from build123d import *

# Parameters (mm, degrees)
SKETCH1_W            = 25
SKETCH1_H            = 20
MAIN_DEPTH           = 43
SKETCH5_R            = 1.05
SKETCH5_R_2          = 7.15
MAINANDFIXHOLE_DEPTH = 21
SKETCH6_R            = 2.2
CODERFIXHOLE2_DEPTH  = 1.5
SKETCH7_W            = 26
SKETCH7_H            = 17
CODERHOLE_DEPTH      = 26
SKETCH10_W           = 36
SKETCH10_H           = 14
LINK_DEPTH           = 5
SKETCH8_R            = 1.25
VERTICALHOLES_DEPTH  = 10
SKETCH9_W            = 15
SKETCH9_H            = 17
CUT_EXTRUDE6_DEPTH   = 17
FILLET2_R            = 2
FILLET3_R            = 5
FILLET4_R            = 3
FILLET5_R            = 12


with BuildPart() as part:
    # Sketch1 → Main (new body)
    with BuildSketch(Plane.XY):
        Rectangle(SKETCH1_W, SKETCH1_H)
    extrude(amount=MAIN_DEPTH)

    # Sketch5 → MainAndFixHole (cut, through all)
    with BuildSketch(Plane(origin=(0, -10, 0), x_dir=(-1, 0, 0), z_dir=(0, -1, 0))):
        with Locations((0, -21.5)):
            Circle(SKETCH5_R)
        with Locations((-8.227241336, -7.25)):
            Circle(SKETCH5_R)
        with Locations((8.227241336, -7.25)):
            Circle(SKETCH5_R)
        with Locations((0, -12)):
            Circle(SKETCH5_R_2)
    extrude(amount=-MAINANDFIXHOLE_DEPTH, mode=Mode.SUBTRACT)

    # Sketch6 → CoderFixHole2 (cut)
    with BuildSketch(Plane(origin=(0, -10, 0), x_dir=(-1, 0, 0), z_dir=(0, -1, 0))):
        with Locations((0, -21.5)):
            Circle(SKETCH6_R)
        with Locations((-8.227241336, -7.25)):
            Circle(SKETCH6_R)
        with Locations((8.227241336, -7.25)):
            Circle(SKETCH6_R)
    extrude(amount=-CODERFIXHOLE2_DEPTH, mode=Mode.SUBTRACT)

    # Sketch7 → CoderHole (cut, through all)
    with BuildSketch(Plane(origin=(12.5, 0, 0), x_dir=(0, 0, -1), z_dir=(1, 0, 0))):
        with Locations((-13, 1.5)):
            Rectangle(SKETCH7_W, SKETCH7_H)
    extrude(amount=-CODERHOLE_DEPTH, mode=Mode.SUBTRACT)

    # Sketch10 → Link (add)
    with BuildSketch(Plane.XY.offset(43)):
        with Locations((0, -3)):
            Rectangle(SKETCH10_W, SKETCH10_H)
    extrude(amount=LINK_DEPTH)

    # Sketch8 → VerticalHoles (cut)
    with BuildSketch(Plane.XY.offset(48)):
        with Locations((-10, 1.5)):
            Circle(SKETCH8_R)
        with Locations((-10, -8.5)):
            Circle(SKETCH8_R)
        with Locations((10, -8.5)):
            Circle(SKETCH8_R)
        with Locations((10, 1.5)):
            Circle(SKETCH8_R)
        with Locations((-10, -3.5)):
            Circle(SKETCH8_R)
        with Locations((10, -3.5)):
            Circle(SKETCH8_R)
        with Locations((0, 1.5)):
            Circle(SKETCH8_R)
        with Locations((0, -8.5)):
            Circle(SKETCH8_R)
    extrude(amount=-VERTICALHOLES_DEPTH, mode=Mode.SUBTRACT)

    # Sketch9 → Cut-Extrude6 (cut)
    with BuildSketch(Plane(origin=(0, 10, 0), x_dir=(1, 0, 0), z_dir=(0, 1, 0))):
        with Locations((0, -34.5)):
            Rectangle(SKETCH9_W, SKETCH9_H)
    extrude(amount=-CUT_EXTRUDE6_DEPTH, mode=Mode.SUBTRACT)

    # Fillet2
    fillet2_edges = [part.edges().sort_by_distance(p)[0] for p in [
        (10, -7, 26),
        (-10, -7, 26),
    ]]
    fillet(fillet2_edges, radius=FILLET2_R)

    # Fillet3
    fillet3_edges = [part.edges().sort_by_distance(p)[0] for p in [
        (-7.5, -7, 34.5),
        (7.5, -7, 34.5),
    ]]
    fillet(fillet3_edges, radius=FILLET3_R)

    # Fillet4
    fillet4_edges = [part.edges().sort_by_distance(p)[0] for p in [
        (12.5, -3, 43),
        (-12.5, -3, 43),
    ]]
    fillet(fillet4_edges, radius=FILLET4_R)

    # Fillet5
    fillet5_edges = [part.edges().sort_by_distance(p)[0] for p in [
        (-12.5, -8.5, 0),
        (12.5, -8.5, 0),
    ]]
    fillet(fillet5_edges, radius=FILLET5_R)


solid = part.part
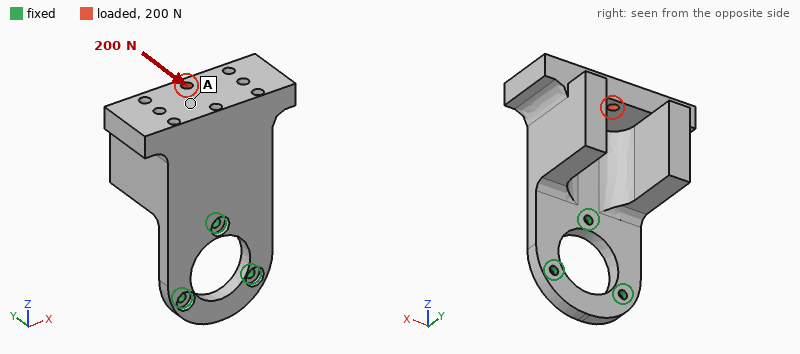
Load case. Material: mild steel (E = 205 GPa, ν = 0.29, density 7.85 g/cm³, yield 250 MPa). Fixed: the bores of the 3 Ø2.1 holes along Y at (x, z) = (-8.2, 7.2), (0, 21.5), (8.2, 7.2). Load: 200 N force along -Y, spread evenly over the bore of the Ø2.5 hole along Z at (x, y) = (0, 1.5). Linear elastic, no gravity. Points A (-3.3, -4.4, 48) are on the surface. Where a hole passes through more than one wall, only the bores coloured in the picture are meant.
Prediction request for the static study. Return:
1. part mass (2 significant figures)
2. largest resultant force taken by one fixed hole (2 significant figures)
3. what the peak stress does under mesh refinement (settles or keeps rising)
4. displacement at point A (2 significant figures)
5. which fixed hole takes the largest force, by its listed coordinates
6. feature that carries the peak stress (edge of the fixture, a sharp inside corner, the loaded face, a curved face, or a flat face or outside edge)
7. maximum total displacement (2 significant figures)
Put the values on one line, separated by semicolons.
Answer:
61 g; 590 N; keeps rising; 0.10 mm; (0, 21.5); edge of the fixture; 0.11 mm
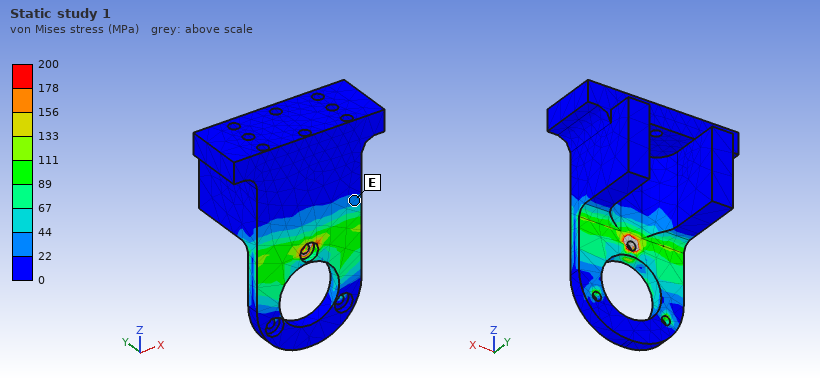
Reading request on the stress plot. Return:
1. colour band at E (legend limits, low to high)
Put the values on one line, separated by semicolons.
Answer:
22 to 44 MPa
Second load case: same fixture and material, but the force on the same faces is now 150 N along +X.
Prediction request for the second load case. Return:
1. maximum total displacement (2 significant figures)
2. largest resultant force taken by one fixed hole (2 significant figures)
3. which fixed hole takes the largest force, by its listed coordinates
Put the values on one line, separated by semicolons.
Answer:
32 µm; 230 N; (0, 21.5)
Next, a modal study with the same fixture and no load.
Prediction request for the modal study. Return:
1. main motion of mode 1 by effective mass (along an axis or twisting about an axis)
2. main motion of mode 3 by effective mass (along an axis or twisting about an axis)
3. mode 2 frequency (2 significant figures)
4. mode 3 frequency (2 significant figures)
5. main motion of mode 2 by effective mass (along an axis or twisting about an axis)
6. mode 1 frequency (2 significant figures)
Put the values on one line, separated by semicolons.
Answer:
along Y; along X; 1800 Hz; 5700 Hz; along X; 1300 Hz
